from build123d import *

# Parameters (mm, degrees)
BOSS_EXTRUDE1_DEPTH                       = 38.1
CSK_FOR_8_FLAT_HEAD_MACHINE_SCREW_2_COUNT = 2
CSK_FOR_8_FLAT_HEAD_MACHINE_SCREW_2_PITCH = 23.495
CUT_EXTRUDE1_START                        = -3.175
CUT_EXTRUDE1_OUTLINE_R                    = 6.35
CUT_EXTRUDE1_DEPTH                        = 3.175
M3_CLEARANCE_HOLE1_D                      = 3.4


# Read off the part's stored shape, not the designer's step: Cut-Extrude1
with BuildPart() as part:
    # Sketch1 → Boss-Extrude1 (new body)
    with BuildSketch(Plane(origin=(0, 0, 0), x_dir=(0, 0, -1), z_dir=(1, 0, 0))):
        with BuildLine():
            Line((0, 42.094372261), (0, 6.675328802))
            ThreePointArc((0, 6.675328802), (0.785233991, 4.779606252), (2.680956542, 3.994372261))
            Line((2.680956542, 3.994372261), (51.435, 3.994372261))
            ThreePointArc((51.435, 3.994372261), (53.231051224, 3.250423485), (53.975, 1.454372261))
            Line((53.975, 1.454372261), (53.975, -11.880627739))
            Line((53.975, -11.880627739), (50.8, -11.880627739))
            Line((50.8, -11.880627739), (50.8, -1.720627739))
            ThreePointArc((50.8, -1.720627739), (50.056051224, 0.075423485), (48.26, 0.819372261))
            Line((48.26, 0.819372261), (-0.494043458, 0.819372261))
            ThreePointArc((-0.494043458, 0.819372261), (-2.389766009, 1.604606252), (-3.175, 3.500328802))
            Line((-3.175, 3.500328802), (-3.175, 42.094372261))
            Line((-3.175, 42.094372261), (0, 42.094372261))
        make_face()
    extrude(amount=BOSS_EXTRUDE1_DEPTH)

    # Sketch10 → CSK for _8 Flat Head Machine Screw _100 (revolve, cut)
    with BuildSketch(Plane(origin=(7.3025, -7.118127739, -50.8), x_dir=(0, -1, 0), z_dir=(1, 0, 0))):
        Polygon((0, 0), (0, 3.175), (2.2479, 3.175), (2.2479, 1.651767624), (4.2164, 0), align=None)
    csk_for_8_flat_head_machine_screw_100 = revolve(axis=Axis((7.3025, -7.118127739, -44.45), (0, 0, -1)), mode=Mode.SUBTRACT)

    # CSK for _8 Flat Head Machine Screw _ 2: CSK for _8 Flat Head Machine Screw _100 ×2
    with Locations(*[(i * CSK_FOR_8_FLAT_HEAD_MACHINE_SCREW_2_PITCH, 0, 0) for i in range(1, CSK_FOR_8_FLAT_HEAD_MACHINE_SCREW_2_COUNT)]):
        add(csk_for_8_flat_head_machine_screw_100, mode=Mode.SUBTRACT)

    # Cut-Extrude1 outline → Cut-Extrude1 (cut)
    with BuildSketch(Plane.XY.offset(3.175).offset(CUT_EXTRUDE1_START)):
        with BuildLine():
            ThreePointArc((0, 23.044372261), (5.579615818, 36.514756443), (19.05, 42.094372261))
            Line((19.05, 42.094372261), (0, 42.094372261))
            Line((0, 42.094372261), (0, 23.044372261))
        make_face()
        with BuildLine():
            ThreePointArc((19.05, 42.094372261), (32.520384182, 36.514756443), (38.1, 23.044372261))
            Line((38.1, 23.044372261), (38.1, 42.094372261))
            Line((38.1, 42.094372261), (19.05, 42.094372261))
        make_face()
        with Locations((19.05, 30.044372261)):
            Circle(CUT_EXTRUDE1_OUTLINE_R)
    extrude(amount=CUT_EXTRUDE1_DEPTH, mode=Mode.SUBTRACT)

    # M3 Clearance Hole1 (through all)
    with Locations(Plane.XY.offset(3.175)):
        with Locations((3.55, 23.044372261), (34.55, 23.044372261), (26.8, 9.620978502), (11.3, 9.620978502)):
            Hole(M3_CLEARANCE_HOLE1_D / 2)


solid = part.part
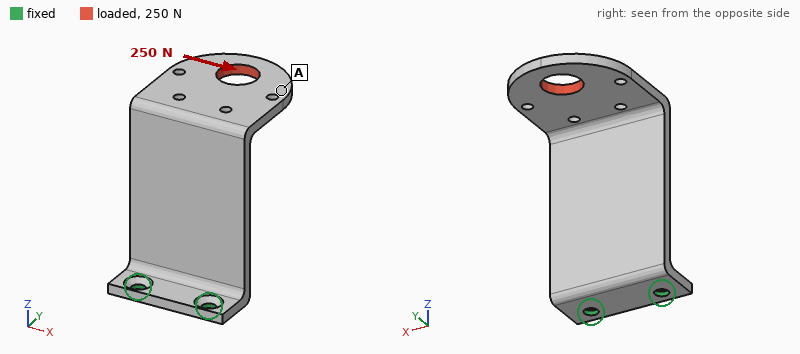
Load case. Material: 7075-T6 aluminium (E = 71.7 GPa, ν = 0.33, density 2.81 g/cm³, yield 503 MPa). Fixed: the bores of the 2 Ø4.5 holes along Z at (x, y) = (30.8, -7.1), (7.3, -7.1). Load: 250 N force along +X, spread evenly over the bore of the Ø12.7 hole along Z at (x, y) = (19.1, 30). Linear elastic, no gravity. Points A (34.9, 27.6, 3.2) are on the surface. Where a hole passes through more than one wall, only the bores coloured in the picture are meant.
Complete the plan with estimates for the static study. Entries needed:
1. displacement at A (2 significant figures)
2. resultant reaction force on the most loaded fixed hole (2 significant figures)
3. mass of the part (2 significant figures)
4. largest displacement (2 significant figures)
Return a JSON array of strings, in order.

["0.78 mm", "670 N", "33 g", "1.0 mm"]
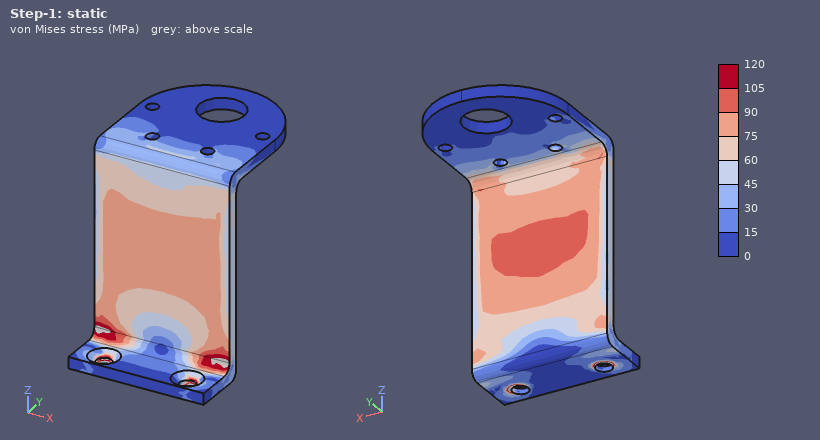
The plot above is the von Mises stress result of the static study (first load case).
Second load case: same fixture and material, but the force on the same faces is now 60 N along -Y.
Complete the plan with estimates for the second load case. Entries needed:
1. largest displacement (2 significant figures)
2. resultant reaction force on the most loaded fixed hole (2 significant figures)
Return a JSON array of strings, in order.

["0.93 mm", "73 N"]
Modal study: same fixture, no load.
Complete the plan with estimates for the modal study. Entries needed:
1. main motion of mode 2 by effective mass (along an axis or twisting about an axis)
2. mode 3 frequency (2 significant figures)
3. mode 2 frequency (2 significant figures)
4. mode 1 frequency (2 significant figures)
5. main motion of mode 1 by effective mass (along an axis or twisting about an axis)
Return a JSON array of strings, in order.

["along X", "1500 Hz", "1000 Hz", "360 Hz", "along Y"]
